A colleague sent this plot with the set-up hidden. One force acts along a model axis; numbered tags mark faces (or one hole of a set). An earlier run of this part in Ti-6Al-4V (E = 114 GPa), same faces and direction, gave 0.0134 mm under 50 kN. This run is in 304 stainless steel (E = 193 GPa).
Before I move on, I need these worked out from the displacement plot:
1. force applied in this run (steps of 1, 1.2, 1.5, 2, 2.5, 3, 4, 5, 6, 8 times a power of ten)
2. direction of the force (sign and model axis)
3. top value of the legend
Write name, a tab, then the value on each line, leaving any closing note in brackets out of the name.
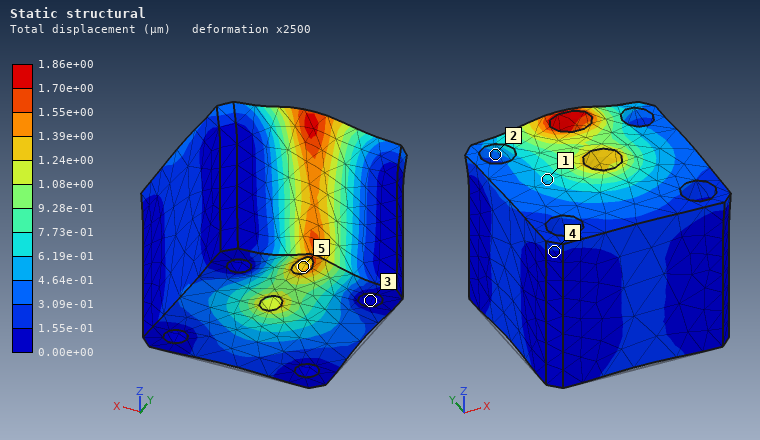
force applied in this run	12 kN
direction of the force	+Z
top value of the legend	1.86e+00 µm
